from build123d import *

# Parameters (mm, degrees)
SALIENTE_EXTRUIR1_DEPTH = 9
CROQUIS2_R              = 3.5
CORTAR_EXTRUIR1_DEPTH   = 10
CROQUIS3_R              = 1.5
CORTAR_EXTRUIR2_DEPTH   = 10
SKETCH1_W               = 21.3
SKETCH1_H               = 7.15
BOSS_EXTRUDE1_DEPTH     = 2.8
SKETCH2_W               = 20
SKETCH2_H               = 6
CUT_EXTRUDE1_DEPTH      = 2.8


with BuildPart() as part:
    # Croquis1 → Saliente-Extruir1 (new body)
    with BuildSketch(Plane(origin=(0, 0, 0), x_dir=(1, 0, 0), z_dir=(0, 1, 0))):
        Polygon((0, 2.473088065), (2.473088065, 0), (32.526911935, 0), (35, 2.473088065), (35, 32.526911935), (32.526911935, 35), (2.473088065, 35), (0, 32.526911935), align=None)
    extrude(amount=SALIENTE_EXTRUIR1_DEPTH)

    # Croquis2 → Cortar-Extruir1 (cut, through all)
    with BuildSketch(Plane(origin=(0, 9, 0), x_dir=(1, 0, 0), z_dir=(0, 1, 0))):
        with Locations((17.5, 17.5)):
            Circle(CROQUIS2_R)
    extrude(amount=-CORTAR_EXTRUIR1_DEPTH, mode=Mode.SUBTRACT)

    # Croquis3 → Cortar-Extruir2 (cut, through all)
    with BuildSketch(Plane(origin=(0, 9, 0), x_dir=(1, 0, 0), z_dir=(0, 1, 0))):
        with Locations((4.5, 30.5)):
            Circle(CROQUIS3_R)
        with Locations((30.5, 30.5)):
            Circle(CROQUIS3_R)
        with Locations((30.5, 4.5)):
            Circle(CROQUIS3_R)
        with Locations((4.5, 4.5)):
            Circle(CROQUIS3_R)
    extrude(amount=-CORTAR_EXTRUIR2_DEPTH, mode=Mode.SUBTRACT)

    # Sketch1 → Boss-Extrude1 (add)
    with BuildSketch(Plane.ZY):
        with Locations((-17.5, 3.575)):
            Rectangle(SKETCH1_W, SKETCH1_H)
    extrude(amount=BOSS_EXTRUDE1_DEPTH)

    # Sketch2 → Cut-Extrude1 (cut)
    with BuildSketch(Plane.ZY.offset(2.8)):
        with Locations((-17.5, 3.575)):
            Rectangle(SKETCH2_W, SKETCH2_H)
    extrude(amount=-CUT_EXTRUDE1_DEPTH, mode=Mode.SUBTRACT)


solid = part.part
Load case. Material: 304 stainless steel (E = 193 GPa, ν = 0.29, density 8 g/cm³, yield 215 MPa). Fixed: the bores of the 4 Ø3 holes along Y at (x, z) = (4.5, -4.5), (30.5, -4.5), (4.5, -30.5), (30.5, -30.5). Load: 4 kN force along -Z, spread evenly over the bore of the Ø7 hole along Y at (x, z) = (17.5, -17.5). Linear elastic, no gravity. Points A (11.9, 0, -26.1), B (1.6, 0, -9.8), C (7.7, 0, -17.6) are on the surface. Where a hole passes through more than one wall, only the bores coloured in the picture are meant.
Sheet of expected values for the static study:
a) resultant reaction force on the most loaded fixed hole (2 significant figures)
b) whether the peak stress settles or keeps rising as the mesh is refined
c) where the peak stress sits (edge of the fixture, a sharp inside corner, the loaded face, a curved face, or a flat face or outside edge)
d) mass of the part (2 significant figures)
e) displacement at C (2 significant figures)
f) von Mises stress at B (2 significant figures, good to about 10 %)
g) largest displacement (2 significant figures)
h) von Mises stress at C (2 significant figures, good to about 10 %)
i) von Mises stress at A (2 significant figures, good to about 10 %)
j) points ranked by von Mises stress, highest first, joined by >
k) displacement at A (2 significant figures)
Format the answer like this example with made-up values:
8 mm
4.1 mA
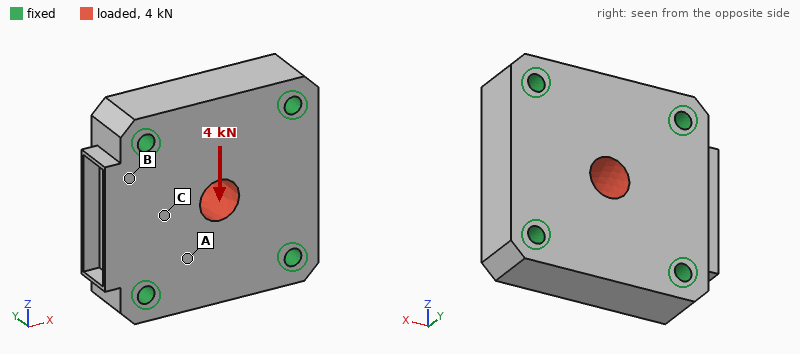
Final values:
1.1 kN
keeps rising
edge of the fixture
83 g
0.55 µm
3.6 MPa
1.6 µm
8.4 MPa
14 MPa
A > C > B
0.84 µm
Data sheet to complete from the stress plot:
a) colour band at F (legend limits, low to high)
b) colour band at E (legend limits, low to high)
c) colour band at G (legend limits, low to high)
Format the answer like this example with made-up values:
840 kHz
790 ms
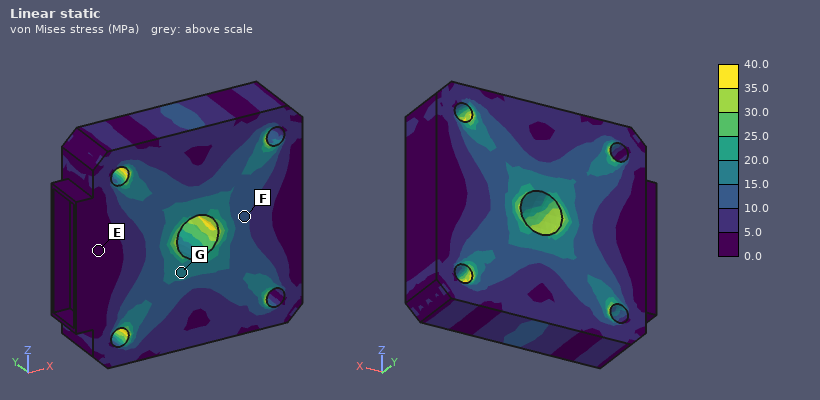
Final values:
10.0 to 15.0 MPa
0.0 to 5.0 MPa
15.0 to 20.0 MPa
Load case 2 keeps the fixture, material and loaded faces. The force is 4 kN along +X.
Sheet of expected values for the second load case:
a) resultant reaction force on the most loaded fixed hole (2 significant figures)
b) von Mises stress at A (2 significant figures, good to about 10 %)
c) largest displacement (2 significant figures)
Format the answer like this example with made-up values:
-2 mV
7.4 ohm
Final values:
1.1 kN
13 MPa
1.6 µm
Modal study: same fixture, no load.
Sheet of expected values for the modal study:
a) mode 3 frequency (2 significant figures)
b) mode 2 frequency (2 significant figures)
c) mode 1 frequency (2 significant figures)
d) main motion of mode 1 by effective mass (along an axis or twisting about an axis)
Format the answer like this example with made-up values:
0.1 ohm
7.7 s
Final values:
45 kHz
43 kHz
31 kHz
along Y
